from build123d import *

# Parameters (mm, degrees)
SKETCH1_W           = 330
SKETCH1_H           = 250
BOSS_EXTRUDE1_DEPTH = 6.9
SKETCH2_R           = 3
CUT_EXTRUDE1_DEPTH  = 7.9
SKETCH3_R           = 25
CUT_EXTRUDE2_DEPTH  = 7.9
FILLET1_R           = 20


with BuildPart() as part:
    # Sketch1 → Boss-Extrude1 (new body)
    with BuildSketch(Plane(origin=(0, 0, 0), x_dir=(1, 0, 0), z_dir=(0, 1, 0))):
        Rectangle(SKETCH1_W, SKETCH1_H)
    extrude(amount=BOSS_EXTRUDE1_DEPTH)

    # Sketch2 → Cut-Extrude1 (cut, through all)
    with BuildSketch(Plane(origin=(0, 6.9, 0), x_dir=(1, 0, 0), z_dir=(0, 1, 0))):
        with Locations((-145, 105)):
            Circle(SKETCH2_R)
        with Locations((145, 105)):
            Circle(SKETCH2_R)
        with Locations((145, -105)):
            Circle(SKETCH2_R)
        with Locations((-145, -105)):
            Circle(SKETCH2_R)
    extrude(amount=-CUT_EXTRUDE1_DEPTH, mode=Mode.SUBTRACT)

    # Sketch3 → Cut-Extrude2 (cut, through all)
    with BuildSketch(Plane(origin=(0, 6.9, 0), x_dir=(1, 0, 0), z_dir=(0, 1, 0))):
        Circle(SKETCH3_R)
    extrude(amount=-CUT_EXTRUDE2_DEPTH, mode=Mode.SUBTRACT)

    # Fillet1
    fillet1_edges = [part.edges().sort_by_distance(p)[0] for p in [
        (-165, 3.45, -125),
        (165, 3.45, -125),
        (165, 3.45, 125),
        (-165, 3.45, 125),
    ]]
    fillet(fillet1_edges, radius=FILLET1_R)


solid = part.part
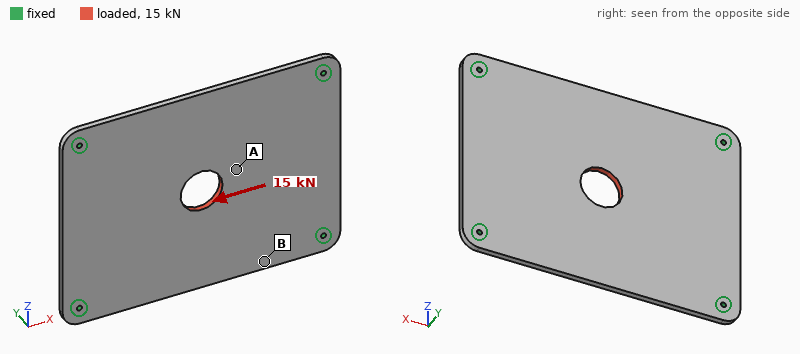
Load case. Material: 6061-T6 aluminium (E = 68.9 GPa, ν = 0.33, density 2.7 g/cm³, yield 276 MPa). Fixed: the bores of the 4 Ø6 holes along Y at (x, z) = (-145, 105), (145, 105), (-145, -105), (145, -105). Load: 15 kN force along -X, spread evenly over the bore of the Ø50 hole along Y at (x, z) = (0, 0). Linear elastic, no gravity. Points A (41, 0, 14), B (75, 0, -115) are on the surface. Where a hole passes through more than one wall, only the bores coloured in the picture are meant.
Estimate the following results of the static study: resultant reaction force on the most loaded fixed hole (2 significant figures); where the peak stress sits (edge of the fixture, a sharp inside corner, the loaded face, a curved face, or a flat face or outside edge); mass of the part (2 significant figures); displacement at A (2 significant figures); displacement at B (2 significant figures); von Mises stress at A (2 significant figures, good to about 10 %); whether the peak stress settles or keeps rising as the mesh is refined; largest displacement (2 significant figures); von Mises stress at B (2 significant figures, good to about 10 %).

4.0 kN
edge of the fixture
1.5 kg
24 µm
10 µm
11 MPa
keeps rising
28 µm
4.9 MPa
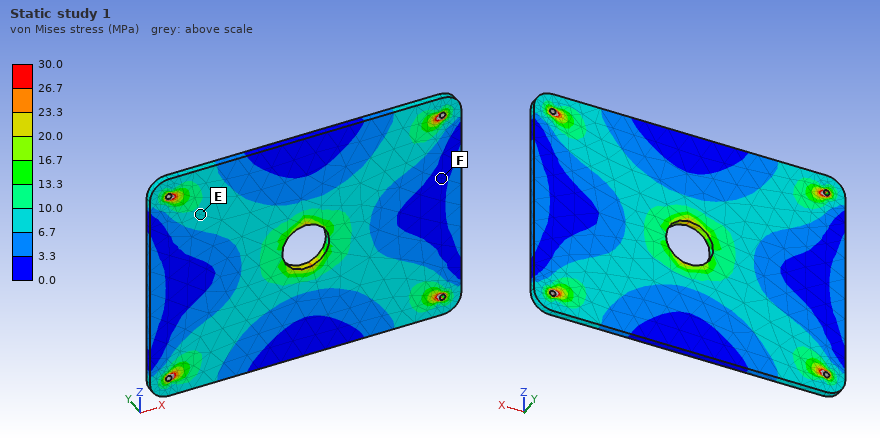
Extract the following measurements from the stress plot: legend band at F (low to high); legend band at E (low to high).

0.0 to 3.3 MPa
6.7 to 10.0 MPa
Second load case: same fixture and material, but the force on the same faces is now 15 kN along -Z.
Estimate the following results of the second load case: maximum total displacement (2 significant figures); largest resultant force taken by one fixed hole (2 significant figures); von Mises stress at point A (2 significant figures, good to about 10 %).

40 µm
4.5 kN
12 MPa
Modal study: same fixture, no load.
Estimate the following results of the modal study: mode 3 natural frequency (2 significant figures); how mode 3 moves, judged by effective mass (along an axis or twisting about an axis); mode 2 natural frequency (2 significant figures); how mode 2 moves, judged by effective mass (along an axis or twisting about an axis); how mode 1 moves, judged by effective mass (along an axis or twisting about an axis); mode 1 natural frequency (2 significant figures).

720 Hz
twisting about Z
510 Hz
twisting about X
along Y
320 Hz
